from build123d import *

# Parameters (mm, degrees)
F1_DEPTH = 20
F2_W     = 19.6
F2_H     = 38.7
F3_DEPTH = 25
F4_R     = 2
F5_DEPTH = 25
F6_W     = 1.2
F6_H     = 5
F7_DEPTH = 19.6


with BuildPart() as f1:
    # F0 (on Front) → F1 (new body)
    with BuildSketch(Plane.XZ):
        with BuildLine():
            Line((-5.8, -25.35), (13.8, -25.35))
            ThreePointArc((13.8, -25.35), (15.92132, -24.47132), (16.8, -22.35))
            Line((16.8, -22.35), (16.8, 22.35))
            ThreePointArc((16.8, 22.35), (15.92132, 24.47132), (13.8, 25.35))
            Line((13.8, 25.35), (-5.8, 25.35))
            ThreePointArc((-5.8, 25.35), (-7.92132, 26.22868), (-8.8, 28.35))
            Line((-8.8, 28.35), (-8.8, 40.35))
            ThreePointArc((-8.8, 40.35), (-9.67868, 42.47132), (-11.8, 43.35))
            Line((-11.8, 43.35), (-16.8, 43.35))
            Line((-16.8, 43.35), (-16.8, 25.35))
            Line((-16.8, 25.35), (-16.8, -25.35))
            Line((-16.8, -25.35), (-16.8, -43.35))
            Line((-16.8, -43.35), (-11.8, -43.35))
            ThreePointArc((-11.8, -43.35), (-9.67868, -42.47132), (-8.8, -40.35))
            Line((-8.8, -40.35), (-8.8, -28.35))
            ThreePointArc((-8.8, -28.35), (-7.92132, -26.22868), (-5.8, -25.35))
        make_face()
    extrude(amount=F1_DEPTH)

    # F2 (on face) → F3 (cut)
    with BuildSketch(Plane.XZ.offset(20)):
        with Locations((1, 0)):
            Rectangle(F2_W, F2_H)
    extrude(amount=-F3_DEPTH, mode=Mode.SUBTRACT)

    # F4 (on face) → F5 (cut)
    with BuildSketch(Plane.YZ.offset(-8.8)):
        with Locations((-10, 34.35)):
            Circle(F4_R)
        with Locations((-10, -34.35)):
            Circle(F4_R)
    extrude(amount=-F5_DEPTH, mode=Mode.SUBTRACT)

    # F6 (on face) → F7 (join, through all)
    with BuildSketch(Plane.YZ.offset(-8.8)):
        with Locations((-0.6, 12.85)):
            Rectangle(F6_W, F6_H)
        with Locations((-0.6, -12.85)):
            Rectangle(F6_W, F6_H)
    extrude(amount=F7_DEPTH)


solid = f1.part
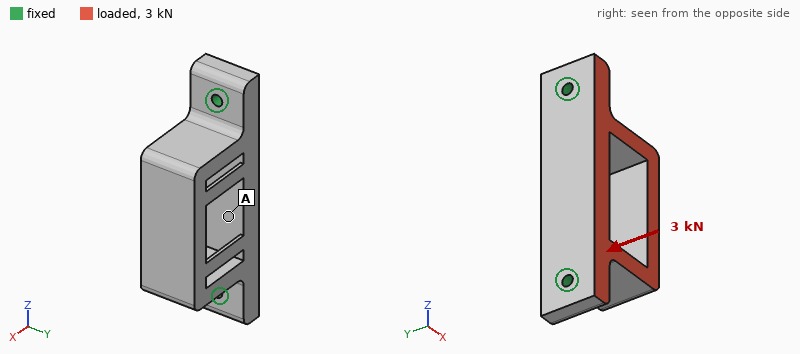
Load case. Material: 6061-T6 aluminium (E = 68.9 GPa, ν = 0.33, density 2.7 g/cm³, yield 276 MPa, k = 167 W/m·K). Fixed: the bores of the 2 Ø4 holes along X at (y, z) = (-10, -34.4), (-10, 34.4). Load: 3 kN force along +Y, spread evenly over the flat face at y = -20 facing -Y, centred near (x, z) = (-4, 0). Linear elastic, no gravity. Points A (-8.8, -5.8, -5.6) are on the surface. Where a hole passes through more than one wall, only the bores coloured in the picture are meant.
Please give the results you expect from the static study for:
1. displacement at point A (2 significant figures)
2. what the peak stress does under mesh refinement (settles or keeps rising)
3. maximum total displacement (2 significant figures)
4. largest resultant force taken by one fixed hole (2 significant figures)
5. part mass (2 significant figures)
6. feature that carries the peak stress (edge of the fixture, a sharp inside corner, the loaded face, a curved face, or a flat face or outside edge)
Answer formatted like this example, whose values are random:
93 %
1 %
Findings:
29 µm
keeps rising
90 µm
1.5 kN
66 g
edge of the fixture
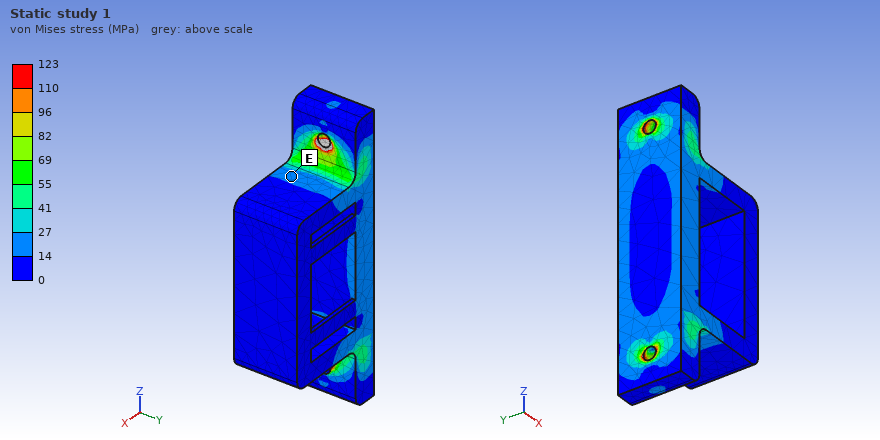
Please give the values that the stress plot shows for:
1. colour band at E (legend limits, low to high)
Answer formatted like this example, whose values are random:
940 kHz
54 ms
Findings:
14 to 27 MPa
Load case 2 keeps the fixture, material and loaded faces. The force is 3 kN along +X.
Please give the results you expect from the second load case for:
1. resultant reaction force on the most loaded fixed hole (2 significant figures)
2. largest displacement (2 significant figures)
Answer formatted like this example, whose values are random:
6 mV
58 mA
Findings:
1.5 kN
84 µm
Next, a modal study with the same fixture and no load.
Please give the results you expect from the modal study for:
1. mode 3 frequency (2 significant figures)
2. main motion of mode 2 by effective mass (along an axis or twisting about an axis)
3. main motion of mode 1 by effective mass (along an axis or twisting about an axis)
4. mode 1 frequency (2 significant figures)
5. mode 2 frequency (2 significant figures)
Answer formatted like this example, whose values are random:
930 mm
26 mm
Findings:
8000 Hz
along Z
along Y
4000 Hz
5800 Hz
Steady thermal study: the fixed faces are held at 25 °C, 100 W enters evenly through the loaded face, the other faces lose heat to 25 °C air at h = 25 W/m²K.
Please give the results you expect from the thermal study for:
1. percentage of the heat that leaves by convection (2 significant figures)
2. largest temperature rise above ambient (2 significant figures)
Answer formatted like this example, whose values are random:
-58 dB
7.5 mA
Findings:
5.1 %
42 K
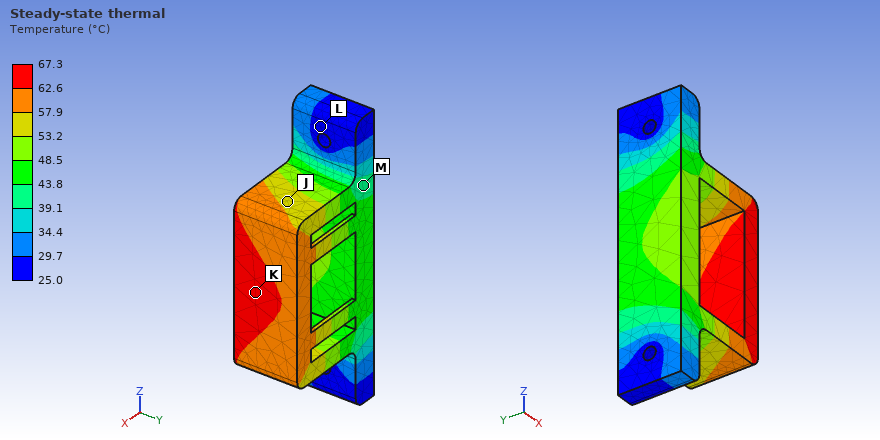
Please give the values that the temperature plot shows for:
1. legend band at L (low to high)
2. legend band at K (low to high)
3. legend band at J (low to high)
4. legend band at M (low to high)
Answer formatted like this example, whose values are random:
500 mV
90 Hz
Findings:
25.0 to 29.7 °C
62.6 to 67.3 °C
53.2 to 57.9 °C
39.1 to 43.8 °C
